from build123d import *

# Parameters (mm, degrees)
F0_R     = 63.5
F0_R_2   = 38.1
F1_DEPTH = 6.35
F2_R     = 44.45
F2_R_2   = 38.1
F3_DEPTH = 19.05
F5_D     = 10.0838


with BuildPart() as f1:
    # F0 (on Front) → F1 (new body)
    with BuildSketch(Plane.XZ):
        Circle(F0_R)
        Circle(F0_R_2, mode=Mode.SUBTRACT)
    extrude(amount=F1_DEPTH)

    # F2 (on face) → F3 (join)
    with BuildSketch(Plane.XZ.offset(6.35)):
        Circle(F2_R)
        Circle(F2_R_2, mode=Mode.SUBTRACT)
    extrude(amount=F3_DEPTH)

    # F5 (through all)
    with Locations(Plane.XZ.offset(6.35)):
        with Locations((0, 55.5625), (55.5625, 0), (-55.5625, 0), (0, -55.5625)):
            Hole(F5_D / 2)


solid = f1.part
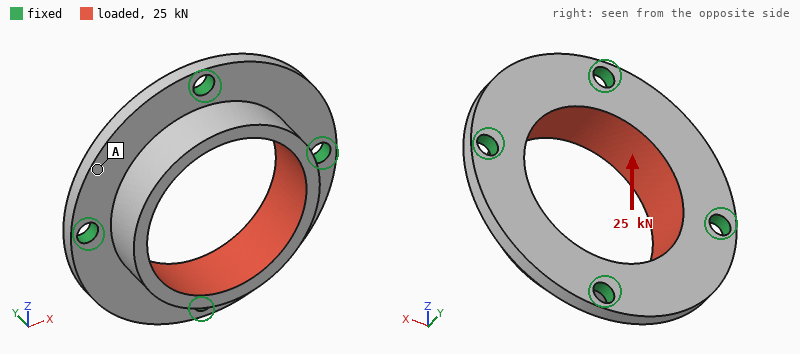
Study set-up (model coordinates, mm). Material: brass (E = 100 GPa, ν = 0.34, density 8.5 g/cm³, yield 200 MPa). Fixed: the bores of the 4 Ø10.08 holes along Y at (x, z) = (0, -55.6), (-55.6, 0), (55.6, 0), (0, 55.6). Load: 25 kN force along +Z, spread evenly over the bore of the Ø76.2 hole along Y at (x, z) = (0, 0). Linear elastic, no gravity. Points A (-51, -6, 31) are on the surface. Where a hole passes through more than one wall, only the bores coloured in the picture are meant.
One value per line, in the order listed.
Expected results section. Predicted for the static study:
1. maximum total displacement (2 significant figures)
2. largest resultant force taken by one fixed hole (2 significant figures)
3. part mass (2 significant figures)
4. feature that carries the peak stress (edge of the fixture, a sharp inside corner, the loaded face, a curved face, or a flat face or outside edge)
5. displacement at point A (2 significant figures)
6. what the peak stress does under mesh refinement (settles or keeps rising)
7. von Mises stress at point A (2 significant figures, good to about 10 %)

34 µm
7.4 kN
690 g
edge of the fixture
18 µm
keeps rising
13 MPa
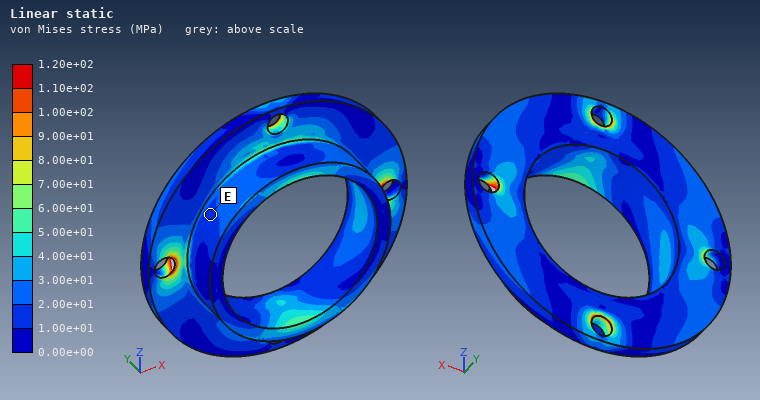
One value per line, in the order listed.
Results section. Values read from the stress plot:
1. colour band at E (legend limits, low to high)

1.00e+01 to 2.00e+01 MPa
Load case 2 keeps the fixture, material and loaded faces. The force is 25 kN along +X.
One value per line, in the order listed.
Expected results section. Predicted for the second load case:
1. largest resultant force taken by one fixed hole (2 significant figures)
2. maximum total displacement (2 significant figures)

7.4 kN
34 µm
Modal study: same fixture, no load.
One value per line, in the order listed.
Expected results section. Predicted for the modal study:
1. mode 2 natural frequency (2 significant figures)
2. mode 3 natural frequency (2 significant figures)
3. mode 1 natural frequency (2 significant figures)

4200 Hz
4200 Hz
3400 Hz
